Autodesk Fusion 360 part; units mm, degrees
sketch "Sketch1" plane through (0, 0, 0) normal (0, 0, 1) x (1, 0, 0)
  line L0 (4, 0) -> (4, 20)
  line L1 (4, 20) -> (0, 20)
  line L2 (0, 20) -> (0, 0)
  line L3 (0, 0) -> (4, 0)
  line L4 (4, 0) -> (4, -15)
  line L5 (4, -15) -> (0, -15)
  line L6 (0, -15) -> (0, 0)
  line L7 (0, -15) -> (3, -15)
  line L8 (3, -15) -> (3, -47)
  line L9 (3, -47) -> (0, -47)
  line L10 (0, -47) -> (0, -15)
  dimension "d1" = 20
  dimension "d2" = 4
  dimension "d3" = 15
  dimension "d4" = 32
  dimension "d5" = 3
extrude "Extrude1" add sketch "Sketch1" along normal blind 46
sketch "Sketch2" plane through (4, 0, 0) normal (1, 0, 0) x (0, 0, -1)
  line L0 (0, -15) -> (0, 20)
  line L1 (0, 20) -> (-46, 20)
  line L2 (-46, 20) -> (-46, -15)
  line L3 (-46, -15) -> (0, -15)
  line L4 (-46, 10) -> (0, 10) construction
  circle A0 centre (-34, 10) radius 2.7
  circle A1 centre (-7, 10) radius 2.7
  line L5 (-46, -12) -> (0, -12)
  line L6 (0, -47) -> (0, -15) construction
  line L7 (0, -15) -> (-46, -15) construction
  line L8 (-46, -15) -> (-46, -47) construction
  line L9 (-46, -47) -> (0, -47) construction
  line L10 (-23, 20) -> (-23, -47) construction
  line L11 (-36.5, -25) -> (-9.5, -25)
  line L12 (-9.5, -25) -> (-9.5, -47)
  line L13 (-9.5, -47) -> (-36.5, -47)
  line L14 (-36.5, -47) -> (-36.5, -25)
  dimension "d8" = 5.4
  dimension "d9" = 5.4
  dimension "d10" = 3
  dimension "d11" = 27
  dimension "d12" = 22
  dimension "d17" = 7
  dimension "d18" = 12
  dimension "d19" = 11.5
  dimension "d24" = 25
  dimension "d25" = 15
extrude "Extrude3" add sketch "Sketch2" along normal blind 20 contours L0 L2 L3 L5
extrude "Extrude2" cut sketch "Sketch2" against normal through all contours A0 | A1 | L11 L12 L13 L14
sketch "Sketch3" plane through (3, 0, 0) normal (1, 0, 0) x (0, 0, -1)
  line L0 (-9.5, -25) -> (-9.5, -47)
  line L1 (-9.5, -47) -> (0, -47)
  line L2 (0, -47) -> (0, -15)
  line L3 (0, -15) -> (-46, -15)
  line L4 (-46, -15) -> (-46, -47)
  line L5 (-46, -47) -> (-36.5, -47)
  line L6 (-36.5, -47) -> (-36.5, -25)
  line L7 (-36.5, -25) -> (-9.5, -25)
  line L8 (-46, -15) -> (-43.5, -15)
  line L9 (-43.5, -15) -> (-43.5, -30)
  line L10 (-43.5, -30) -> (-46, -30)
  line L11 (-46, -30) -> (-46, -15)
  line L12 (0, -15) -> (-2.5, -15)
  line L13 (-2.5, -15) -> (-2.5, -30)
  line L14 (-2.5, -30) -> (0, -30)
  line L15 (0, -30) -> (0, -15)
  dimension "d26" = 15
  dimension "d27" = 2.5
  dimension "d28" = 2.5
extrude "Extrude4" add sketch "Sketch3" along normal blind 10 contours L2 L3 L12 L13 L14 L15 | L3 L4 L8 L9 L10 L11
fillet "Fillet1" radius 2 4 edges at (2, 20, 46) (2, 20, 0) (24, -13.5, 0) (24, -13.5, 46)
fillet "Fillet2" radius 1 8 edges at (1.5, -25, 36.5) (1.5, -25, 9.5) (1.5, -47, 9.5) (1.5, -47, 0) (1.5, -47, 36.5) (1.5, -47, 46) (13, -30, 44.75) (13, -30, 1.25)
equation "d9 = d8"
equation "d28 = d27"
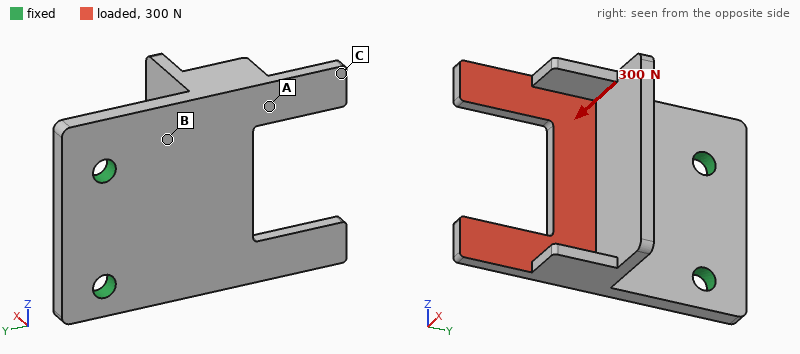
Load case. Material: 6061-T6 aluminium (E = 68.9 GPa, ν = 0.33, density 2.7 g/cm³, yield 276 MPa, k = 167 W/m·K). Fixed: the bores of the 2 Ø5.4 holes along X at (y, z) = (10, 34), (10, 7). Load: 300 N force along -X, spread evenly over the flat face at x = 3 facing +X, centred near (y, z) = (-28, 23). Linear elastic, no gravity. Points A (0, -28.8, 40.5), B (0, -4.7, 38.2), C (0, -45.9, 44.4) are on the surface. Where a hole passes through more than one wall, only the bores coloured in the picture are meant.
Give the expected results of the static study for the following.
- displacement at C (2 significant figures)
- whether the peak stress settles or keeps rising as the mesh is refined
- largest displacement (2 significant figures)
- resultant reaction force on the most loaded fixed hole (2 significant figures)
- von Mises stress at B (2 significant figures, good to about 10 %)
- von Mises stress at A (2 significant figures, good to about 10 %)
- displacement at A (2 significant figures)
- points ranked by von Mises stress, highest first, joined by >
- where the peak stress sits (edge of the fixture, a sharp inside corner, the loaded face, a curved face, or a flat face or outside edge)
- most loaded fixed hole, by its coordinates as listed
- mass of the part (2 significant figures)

0.56 mm
keeps rising
0.58 mm
170 N
52 MPa
33 MPa
0.31 mm
B > A > C
edge of the fixture
(10, 34)
33 g
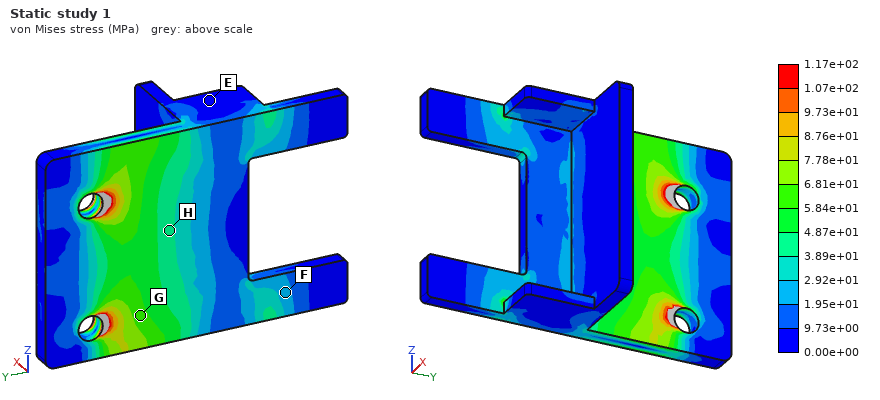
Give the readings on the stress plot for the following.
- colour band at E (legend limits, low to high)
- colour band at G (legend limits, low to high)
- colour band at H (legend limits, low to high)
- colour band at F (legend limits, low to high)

0.00e+00 to 9.73e+00 MPa
5.84e+01 to 6.81e+01 MPa
3.89e+01 to 4.87e+01 MPa
1.95e+01 to 2.92e+01 MPa
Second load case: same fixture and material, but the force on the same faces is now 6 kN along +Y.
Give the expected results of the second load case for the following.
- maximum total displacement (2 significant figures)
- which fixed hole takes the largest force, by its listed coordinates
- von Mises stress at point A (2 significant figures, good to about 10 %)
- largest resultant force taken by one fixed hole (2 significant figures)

0.62 mm
(10, 34)
68 MPa
3.5 kN
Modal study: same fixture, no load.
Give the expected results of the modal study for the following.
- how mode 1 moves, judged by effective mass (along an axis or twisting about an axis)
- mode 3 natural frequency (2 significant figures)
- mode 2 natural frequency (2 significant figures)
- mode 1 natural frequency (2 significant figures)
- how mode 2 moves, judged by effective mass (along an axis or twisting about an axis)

along X
5300 Hz
2200 Hz
1400 Hz
twisting about Y
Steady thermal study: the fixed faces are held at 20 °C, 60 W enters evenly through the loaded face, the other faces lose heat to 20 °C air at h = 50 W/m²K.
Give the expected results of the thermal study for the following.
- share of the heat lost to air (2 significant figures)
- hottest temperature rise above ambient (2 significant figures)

21 %
88 K
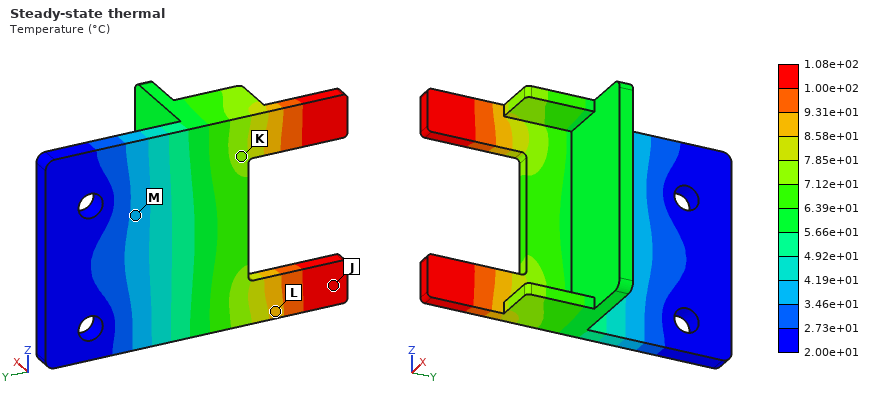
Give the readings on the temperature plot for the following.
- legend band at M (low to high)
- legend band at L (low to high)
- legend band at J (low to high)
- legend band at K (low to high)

3.46e+01 to 4.19e+01 °C
8.58e+01 to 9.31e+01 °C
1.00e+02 to 1.08e+02 °C
7.12e+01 to 7.85e+01 °C
